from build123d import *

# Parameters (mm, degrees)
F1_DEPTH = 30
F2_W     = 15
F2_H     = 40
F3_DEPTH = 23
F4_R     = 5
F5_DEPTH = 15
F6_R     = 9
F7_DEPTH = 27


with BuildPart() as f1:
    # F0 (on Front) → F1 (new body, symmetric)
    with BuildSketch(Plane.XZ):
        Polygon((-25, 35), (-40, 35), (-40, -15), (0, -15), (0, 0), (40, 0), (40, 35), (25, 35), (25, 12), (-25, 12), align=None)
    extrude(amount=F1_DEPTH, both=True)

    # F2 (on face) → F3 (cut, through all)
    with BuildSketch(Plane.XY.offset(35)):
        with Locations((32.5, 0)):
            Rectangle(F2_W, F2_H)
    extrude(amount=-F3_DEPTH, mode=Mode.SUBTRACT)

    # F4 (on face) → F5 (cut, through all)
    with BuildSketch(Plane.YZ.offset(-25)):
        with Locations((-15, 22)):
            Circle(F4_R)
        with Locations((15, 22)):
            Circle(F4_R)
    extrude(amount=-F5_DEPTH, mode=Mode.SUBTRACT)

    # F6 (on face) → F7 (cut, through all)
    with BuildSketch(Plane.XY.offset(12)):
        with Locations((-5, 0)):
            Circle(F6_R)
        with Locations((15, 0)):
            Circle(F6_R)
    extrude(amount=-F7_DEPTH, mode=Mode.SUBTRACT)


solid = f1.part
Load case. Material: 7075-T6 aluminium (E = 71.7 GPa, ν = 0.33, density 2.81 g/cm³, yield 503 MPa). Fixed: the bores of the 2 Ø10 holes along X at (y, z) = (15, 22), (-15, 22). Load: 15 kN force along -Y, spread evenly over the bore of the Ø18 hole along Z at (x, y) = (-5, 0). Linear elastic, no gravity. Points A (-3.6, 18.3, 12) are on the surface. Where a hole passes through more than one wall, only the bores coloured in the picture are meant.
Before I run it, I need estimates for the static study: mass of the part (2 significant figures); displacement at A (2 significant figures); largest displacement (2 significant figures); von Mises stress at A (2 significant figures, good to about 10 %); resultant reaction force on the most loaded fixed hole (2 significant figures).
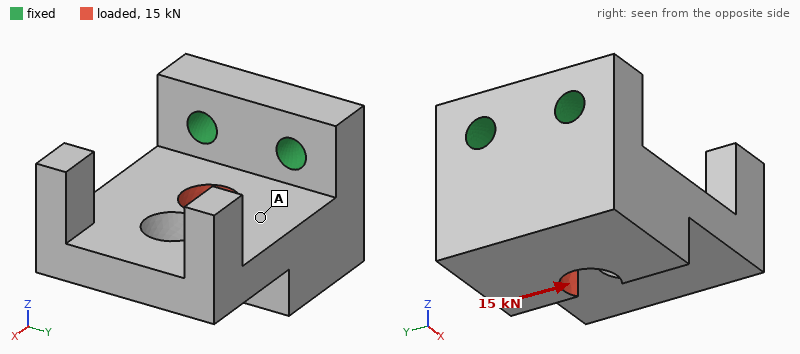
310 g
0.065 mm
0.14 mm
27 MPa
14 kN
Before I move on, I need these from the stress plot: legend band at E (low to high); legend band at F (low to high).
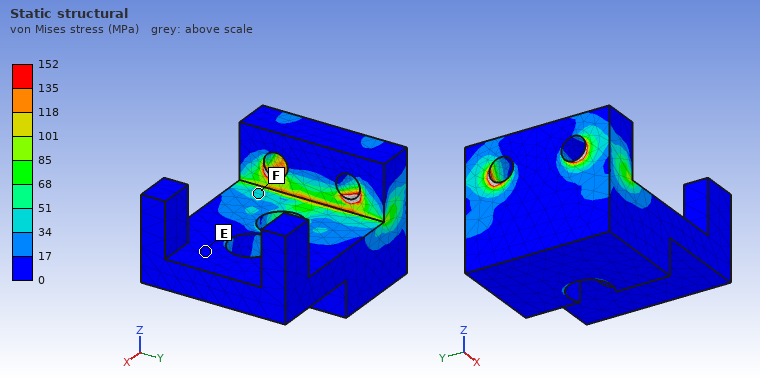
0 to 17 MPa
34 to 51 MPa
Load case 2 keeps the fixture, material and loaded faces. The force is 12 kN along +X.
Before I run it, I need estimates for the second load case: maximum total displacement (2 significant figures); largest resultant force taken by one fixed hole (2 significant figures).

0.16 mm
6.0 kN
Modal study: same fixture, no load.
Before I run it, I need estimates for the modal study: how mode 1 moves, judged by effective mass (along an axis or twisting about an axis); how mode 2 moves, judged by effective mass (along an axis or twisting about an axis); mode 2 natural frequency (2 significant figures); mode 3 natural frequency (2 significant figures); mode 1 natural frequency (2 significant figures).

along Z
along Y
3200 Hz
4300 Hz
1800 Hz
